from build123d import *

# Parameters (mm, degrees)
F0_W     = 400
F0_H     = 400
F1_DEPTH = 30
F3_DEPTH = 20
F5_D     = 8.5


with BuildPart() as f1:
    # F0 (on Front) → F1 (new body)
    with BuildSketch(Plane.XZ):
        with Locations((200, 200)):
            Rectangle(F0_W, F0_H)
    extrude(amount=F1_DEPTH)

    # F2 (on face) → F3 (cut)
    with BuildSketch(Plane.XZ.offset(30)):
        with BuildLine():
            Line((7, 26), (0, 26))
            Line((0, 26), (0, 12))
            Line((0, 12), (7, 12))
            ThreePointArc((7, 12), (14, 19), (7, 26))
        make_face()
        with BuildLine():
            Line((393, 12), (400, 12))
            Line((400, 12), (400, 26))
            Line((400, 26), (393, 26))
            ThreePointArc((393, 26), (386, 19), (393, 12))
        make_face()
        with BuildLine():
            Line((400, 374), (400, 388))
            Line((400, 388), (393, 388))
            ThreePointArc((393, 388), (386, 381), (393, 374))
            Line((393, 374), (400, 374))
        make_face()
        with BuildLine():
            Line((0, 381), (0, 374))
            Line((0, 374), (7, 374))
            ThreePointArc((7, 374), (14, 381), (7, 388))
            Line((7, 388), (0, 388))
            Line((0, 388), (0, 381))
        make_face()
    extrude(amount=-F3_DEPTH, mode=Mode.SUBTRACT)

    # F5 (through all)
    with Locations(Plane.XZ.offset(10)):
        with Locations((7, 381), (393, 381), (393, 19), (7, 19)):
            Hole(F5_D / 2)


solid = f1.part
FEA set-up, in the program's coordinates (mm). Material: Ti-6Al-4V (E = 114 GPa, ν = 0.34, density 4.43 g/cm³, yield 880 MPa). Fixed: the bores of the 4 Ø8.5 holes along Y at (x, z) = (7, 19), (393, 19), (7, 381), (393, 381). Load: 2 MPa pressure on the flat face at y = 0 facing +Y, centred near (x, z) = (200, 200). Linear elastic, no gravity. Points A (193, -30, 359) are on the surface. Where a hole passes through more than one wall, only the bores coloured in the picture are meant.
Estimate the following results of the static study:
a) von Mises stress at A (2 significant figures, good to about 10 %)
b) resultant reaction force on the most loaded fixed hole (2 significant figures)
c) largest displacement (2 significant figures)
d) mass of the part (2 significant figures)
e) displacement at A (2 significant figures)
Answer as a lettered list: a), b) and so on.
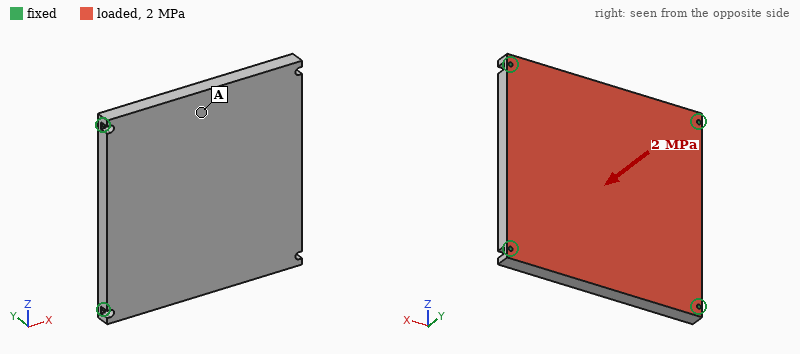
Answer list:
a) 200 MPa
b) 170 kN
c) 2.3 mm
d) 21 kg
e) 1.8 mm
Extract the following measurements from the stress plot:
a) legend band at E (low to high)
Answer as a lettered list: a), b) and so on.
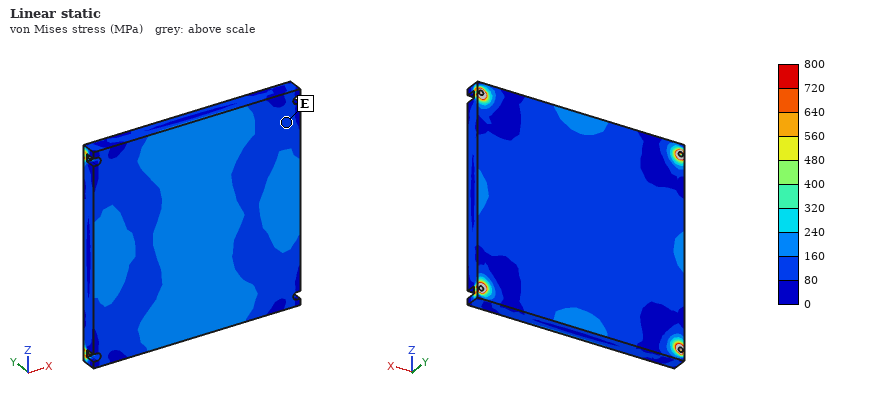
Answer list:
a) 80 to 160 MPa
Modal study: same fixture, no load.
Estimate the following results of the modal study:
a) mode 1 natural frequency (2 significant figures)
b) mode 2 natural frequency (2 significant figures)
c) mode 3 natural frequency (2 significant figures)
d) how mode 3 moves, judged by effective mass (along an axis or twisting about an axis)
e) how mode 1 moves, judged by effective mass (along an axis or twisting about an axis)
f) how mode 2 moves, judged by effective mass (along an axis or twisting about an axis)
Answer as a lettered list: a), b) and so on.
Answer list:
a) 470 Hz
b) 840 Hz
c) 910 Hz
d) twisting about Z
e) along Y
f) twisting about X
